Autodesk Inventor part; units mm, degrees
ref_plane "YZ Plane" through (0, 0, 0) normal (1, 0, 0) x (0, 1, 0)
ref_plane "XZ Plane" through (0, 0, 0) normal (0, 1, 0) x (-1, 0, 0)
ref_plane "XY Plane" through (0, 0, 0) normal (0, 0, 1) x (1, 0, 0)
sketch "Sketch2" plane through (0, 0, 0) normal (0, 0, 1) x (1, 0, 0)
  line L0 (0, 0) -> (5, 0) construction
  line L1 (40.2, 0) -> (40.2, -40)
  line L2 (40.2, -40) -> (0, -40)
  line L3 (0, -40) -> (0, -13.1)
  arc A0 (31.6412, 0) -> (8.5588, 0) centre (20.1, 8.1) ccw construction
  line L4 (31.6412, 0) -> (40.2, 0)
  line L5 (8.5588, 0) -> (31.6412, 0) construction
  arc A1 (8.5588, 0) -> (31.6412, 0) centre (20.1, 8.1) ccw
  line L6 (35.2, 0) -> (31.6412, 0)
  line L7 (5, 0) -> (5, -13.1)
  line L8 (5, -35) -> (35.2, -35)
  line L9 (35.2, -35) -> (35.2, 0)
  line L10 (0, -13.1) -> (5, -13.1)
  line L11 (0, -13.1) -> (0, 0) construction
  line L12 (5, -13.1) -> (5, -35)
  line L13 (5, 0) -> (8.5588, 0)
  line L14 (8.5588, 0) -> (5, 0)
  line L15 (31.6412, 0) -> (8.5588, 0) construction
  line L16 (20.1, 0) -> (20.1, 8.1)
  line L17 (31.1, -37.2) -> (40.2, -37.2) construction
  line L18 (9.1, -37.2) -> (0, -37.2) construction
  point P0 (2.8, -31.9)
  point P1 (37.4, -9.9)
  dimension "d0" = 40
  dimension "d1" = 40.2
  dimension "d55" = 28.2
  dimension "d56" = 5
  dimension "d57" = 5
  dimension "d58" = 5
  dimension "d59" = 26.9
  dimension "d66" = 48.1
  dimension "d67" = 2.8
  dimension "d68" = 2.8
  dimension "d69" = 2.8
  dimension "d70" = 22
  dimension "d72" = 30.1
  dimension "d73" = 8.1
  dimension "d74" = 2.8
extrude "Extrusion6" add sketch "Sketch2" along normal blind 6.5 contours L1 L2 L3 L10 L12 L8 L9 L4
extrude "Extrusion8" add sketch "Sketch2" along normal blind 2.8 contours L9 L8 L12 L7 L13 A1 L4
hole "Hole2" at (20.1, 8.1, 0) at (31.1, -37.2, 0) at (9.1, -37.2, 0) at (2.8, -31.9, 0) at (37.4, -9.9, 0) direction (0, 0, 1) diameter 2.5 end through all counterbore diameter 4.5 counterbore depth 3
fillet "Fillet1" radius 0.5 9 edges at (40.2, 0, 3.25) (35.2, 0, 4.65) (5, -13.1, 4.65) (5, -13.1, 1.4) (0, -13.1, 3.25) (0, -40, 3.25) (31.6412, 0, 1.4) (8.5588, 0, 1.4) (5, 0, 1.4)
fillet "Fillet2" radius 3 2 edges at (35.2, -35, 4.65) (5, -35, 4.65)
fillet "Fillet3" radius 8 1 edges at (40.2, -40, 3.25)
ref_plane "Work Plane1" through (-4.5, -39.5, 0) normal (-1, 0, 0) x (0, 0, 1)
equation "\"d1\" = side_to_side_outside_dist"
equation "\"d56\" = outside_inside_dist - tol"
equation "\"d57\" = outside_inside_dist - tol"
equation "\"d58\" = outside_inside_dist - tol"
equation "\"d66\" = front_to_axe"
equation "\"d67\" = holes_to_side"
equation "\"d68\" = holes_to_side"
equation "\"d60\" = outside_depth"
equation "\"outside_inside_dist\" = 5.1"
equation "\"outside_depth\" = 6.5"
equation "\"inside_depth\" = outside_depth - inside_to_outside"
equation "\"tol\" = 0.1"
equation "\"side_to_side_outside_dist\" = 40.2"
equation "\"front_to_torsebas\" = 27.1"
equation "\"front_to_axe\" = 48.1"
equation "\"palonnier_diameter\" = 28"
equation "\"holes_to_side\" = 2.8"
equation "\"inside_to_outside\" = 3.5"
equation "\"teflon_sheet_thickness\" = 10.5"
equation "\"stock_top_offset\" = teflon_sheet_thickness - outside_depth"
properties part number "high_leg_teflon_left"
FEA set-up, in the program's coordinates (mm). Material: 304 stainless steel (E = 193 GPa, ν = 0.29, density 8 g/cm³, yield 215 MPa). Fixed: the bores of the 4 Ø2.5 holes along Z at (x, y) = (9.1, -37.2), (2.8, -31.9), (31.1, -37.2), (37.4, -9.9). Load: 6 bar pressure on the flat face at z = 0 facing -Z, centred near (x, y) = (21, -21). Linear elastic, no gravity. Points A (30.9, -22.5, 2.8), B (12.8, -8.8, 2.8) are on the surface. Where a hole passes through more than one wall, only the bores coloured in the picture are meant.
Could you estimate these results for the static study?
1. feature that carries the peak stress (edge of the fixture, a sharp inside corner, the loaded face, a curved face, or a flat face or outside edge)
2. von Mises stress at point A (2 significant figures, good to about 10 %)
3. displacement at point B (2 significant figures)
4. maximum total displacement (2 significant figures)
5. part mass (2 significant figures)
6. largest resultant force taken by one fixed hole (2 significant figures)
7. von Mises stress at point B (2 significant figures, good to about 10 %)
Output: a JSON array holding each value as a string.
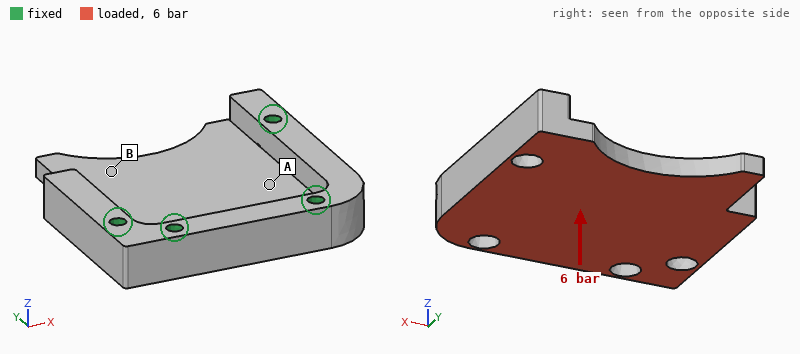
["a curved face", "13 MPa", "24 µm", "39 µm", "44 g", "490 N", "27 MPa"]
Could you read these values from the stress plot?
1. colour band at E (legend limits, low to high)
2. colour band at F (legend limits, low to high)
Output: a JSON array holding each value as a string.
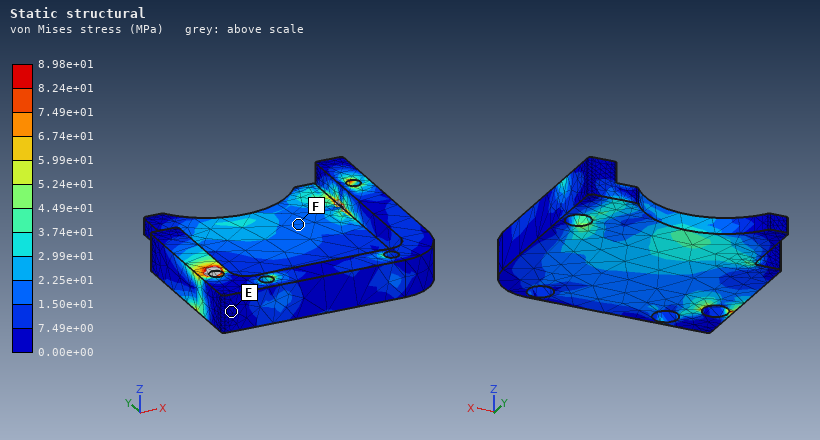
["0.00e+00 to 7.49e+00 MPa", "1.50e+01 to 2.25e+01 MPa"]
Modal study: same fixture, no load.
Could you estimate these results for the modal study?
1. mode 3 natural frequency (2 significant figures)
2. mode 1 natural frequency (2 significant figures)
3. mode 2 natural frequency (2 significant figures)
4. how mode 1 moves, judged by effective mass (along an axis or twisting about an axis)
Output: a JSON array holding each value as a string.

["15 kHz", "6000 Hz", "13 kHz", "along Z"]
